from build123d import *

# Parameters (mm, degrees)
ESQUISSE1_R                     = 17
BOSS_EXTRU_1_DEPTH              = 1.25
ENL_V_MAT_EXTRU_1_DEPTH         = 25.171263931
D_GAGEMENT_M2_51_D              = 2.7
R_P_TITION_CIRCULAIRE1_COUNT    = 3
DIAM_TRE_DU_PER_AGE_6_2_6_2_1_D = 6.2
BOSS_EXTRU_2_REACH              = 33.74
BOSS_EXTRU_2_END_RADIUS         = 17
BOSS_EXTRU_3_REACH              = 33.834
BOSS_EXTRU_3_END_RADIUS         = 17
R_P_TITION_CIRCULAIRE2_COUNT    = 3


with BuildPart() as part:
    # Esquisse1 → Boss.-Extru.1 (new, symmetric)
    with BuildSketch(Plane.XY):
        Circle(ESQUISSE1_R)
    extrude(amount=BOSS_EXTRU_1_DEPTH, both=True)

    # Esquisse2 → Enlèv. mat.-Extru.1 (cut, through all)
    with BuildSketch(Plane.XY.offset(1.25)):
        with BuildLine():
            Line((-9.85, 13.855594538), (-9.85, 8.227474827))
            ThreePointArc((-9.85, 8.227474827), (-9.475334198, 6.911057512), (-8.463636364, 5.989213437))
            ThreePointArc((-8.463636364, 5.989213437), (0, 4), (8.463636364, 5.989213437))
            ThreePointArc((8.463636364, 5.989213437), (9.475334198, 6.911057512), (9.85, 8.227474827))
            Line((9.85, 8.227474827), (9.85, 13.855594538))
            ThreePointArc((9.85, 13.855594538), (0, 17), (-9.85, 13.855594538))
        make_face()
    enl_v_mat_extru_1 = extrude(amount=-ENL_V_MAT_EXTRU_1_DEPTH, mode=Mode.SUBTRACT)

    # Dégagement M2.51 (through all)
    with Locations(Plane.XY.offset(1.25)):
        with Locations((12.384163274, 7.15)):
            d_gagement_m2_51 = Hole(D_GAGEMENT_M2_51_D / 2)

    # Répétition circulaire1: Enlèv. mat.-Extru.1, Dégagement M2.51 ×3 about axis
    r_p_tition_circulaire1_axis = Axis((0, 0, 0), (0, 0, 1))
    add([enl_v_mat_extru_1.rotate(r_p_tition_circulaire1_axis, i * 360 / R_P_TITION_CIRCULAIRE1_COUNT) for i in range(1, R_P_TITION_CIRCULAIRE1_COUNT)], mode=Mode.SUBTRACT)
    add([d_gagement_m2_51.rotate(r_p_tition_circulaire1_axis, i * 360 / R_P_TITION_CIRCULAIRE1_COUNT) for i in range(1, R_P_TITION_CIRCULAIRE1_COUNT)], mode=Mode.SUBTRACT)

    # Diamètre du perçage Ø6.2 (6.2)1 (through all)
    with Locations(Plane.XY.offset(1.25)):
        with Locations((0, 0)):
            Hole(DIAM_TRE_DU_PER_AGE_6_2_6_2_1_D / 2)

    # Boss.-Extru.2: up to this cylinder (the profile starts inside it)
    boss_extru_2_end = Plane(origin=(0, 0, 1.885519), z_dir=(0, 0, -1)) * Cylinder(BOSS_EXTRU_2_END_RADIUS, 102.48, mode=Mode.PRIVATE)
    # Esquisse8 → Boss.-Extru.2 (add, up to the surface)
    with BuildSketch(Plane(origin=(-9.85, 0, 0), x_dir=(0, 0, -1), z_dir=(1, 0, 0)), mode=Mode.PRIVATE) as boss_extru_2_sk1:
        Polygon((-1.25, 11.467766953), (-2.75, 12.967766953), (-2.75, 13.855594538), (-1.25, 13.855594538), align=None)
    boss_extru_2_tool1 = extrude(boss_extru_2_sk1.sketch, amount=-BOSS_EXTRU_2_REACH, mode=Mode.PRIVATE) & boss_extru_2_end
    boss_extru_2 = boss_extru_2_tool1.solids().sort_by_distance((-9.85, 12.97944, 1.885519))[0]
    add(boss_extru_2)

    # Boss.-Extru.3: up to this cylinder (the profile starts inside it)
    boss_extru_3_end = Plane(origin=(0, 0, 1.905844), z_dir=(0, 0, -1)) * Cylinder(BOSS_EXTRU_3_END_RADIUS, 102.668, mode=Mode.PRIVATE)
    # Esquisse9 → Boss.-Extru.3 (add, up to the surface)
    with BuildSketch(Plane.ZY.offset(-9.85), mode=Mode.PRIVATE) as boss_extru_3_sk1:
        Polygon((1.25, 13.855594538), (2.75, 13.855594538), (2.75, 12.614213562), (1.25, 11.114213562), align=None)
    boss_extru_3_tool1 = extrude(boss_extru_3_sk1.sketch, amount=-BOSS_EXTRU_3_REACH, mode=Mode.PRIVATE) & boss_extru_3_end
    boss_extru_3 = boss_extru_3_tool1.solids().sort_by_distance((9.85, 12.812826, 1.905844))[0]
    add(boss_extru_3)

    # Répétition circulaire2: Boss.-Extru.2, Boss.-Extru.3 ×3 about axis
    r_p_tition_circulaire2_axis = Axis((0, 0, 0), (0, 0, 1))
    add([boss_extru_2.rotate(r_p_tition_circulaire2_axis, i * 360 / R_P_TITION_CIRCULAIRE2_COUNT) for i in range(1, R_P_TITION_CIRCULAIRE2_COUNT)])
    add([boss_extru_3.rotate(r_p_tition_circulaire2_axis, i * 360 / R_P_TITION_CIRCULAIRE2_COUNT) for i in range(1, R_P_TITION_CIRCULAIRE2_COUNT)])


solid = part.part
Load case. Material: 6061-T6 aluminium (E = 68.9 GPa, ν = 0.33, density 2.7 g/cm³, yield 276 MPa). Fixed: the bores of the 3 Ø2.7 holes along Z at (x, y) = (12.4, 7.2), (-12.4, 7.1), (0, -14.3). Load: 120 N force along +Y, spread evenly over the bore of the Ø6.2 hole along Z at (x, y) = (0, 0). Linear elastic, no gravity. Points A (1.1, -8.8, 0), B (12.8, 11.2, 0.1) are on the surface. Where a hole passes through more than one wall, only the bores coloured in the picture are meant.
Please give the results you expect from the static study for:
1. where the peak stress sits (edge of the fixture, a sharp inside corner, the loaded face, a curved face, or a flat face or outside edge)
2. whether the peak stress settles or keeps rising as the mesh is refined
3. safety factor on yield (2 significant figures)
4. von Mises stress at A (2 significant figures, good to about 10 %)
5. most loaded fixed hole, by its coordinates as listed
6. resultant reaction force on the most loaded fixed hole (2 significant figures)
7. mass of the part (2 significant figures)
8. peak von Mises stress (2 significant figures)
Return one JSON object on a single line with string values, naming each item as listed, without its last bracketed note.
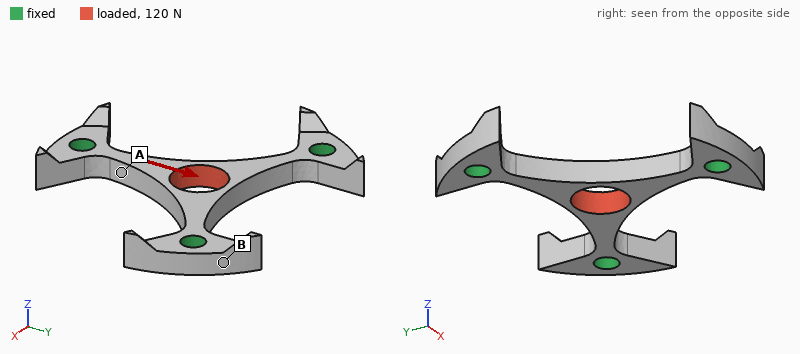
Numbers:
{"where the peak stress sits": "the loaded face", "whether the peak stress settles or keeps rising as the mesh is refined": "settles", "safety factor on yield": "5.5", "von Mises stress at A": "15 MPa", "most loaded fixed hole, by its coordinates as listed": "(0, -14.3)", "resultant reaction force on the most loaded fixed hole": "81 N", "mass of the part": "1.4 g", "peak von Mises stress": "50 MPa"}
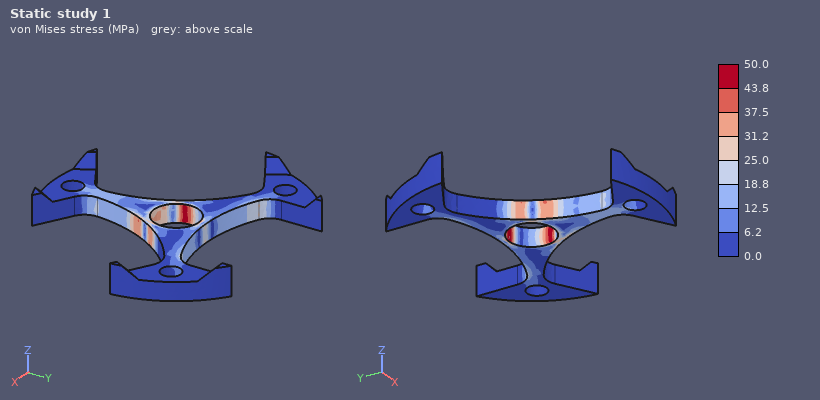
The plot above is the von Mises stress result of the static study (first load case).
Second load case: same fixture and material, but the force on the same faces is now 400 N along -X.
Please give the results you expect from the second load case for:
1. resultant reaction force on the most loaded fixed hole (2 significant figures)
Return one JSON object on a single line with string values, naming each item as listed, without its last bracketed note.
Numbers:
{"resultant reaction force on the most loaded fixed hole": "230 N"}
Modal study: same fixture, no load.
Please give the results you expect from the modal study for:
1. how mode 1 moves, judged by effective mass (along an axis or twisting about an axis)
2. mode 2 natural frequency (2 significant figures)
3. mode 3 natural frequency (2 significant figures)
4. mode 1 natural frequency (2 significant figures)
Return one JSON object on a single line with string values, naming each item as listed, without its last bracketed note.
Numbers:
{"how mode 1 moves, judged by effective mass": "along Z", "mode 2 natural frequency": "36 kHz", "mode 3 natural frequency": "36 kHz", "mode 1 natural frequency": "18 kHz"}
